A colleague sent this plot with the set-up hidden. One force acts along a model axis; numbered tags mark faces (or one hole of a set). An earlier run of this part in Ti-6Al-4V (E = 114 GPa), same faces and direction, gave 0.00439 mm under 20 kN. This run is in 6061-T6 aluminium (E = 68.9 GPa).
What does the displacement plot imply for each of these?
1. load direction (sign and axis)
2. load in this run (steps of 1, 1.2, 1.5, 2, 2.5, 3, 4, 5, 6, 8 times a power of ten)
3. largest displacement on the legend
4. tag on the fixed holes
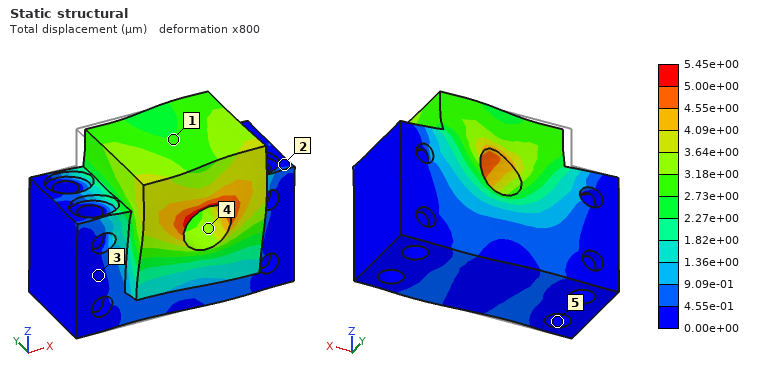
+X
15 kN
5.45e+00 µm
5
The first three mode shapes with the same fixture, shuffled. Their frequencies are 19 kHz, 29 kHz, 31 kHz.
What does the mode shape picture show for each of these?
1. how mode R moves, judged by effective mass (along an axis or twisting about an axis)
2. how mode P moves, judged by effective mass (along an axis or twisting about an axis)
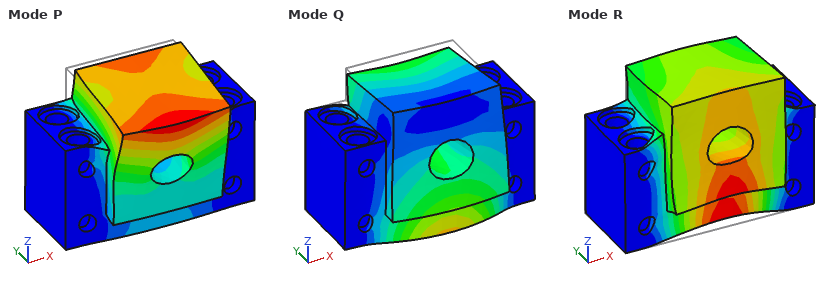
along Z
along Y
